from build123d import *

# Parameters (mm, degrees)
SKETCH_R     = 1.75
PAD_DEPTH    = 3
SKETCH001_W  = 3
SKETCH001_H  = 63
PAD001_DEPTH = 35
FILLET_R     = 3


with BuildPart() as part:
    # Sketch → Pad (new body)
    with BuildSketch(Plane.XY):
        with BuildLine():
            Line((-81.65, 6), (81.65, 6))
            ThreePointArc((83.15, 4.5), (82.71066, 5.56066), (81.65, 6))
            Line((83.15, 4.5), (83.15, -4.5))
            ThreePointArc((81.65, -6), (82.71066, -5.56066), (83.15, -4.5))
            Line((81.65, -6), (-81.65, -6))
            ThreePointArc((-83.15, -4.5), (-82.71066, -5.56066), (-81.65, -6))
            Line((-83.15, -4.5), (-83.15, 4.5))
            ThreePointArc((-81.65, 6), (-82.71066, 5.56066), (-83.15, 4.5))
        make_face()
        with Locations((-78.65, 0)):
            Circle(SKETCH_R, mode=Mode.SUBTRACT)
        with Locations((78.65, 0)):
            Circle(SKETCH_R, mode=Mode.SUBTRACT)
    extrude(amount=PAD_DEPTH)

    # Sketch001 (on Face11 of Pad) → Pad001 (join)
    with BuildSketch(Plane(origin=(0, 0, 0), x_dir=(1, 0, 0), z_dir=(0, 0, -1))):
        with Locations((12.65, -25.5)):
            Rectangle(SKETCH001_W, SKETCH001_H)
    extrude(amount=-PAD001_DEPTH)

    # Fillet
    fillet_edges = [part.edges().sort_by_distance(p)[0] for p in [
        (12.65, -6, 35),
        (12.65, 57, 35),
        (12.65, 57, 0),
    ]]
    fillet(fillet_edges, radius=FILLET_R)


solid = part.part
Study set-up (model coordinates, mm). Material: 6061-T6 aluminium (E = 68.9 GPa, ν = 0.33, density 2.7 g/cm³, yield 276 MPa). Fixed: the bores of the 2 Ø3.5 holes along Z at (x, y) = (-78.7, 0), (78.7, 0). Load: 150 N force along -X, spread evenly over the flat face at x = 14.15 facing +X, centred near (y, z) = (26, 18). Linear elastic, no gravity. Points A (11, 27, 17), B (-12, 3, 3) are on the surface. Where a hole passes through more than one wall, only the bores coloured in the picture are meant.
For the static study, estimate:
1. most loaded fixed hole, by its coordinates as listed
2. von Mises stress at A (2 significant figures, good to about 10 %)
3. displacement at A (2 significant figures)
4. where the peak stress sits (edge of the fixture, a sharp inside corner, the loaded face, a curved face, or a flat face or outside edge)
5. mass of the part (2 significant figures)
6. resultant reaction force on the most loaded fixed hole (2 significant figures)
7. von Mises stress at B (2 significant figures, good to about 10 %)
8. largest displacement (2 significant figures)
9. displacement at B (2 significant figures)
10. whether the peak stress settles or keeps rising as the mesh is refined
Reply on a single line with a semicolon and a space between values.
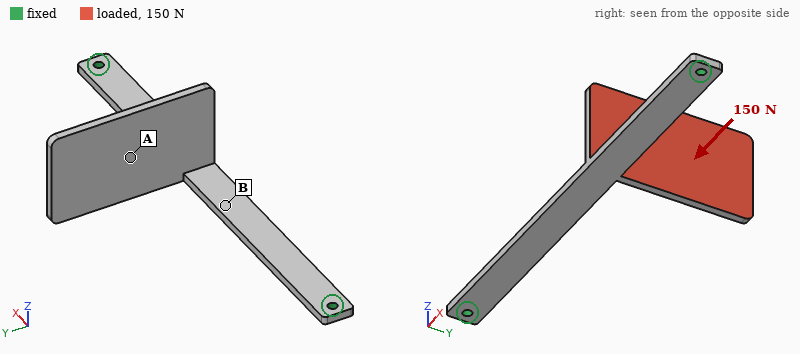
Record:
(78.7, 0); 20 MPa; 0.65 mm; a sharp inside corner; 34 g; 95 N; 52 MPa; 1.6 mm; 0.30 mm; keeps rising
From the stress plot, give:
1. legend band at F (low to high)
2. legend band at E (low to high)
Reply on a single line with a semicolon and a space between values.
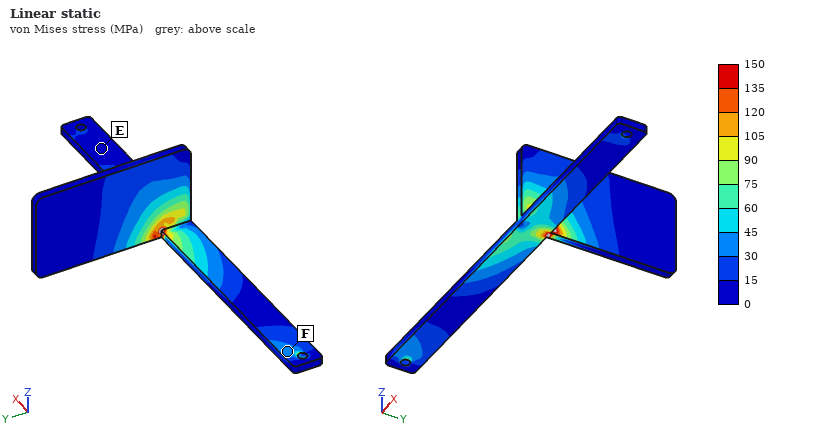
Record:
30 to 45 MPa; 0 to 15 MPa
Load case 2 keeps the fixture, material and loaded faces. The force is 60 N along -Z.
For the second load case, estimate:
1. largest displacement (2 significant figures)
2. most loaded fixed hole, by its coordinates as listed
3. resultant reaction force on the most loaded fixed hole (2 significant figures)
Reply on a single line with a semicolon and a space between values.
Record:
2.1 mm; (78.7, 0); 38 N
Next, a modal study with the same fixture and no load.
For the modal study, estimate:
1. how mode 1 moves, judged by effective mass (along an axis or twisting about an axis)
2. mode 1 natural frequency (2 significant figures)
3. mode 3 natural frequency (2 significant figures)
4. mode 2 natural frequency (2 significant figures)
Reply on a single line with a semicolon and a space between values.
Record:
along Z; 230 Hz; 530 Hz; 450 Hz
